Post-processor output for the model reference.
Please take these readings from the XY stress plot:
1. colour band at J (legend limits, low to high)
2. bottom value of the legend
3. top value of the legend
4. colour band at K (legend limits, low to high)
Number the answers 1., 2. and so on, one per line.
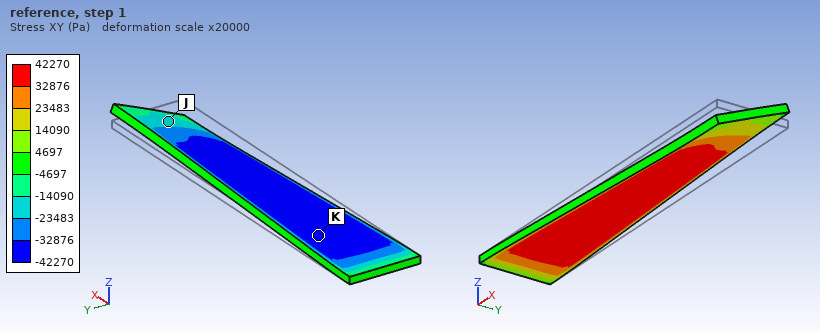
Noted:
1. -23483 to -14090 Pa
2. -42270 Pa
3. 42270 Pa
4. -42270 to -32876 Pa
